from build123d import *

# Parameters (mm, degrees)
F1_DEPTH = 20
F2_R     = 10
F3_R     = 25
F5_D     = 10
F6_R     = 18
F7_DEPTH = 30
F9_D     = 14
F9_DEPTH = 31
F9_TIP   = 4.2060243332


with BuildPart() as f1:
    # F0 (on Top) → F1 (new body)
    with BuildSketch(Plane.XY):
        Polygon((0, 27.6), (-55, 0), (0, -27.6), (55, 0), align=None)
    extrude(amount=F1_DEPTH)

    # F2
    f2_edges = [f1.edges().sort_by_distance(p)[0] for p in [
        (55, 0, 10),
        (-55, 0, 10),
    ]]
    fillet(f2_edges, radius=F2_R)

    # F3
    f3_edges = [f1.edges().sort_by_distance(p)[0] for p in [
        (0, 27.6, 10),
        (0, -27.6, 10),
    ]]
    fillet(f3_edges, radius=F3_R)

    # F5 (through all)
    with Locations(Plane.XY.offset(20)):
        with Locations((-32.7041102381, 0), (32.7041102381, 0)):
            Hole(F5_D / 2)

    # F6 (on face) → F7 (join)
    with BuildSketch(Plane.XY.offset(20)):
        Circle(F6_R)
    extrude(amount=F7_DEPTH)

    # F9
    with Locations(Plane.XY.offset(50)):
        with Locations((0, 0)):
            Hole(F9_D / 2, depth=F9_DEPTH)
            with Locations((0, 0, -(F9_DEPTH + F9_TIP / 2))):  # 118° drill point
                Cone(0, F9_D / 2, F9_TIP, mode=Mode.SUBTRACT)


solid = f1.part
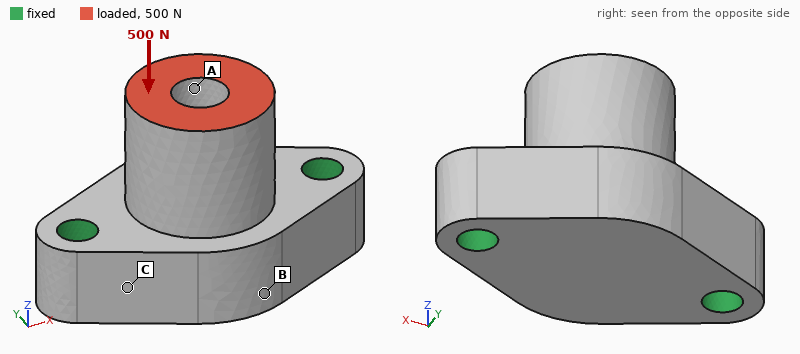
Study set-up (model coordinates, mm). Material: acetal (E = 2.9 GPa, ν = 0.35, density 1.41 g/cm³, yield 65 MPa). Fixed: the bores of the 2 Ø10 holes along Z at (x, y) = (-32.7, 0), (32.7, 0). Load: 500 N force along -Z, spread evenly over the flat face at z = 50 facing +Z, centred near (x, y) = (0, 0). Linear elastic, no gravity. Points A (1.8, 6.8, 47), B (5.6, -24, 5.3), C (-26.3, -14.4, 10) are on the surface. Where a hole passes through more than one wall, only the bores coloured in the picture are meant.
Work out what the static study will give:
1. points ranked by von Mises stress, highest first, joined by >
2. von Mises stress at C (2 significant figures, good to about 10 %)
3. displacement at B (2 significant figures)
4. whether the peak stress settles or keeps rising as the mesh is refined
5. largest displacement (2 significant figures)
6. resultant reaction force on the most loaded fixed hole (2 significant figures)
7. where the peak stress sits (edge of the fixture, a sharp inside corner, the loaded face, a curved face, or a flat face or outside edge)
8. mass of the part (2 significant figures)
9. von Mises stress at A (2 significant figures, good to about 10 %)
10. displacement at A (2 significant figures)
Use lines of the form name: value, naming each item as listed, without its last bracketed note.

points ranked by von Mises stress, highest first, joined by >: C > A > B
von Mises stress at C: 0.76 MPa
displacement at B: 14 µm
whether the peak stress settles or keeps rising as the mesh is refined: keeps rising
largest displacement: 18 µm
resultant reaction force on the most loaded fixed hole: 250 N
where the peak stress sits: edge of the fixture
mass of the part: 110 g
von Mises stress at A: 0.54 MPa
displacement at A: 18 µm
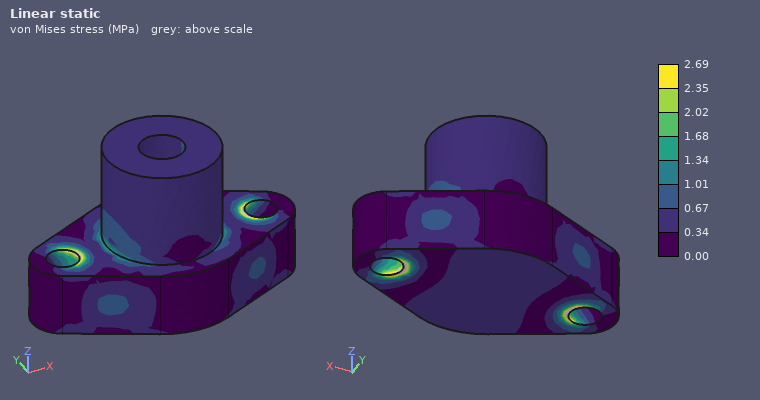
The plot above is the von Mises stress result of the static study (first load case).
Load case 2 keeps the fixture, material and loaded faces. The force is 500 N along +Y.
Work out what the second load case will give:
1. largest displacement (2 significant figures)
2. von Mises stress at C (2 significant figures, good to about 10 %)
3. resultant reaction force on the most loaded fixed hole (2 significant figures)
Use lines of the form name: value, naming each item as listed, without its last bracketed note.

largest displacement: 0.22 mm
von Mises stress at C: 4.6 MPa
resultant reaction force on the most loaded fixed hole: 250 N
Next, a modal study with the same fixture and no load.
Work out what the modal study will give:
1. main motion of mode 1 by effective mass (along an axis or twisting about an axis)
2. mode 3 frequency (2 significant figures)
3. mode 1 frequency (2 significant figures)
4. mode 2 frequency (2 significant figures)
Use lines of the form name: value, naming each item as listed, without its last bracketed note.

main motion of mode 1 by effective mass: along Y
mode 3 frequency: 3400 Hz
mode 1 frequency: 1800 Hz
mode 2 frequency: 3300 Hz
